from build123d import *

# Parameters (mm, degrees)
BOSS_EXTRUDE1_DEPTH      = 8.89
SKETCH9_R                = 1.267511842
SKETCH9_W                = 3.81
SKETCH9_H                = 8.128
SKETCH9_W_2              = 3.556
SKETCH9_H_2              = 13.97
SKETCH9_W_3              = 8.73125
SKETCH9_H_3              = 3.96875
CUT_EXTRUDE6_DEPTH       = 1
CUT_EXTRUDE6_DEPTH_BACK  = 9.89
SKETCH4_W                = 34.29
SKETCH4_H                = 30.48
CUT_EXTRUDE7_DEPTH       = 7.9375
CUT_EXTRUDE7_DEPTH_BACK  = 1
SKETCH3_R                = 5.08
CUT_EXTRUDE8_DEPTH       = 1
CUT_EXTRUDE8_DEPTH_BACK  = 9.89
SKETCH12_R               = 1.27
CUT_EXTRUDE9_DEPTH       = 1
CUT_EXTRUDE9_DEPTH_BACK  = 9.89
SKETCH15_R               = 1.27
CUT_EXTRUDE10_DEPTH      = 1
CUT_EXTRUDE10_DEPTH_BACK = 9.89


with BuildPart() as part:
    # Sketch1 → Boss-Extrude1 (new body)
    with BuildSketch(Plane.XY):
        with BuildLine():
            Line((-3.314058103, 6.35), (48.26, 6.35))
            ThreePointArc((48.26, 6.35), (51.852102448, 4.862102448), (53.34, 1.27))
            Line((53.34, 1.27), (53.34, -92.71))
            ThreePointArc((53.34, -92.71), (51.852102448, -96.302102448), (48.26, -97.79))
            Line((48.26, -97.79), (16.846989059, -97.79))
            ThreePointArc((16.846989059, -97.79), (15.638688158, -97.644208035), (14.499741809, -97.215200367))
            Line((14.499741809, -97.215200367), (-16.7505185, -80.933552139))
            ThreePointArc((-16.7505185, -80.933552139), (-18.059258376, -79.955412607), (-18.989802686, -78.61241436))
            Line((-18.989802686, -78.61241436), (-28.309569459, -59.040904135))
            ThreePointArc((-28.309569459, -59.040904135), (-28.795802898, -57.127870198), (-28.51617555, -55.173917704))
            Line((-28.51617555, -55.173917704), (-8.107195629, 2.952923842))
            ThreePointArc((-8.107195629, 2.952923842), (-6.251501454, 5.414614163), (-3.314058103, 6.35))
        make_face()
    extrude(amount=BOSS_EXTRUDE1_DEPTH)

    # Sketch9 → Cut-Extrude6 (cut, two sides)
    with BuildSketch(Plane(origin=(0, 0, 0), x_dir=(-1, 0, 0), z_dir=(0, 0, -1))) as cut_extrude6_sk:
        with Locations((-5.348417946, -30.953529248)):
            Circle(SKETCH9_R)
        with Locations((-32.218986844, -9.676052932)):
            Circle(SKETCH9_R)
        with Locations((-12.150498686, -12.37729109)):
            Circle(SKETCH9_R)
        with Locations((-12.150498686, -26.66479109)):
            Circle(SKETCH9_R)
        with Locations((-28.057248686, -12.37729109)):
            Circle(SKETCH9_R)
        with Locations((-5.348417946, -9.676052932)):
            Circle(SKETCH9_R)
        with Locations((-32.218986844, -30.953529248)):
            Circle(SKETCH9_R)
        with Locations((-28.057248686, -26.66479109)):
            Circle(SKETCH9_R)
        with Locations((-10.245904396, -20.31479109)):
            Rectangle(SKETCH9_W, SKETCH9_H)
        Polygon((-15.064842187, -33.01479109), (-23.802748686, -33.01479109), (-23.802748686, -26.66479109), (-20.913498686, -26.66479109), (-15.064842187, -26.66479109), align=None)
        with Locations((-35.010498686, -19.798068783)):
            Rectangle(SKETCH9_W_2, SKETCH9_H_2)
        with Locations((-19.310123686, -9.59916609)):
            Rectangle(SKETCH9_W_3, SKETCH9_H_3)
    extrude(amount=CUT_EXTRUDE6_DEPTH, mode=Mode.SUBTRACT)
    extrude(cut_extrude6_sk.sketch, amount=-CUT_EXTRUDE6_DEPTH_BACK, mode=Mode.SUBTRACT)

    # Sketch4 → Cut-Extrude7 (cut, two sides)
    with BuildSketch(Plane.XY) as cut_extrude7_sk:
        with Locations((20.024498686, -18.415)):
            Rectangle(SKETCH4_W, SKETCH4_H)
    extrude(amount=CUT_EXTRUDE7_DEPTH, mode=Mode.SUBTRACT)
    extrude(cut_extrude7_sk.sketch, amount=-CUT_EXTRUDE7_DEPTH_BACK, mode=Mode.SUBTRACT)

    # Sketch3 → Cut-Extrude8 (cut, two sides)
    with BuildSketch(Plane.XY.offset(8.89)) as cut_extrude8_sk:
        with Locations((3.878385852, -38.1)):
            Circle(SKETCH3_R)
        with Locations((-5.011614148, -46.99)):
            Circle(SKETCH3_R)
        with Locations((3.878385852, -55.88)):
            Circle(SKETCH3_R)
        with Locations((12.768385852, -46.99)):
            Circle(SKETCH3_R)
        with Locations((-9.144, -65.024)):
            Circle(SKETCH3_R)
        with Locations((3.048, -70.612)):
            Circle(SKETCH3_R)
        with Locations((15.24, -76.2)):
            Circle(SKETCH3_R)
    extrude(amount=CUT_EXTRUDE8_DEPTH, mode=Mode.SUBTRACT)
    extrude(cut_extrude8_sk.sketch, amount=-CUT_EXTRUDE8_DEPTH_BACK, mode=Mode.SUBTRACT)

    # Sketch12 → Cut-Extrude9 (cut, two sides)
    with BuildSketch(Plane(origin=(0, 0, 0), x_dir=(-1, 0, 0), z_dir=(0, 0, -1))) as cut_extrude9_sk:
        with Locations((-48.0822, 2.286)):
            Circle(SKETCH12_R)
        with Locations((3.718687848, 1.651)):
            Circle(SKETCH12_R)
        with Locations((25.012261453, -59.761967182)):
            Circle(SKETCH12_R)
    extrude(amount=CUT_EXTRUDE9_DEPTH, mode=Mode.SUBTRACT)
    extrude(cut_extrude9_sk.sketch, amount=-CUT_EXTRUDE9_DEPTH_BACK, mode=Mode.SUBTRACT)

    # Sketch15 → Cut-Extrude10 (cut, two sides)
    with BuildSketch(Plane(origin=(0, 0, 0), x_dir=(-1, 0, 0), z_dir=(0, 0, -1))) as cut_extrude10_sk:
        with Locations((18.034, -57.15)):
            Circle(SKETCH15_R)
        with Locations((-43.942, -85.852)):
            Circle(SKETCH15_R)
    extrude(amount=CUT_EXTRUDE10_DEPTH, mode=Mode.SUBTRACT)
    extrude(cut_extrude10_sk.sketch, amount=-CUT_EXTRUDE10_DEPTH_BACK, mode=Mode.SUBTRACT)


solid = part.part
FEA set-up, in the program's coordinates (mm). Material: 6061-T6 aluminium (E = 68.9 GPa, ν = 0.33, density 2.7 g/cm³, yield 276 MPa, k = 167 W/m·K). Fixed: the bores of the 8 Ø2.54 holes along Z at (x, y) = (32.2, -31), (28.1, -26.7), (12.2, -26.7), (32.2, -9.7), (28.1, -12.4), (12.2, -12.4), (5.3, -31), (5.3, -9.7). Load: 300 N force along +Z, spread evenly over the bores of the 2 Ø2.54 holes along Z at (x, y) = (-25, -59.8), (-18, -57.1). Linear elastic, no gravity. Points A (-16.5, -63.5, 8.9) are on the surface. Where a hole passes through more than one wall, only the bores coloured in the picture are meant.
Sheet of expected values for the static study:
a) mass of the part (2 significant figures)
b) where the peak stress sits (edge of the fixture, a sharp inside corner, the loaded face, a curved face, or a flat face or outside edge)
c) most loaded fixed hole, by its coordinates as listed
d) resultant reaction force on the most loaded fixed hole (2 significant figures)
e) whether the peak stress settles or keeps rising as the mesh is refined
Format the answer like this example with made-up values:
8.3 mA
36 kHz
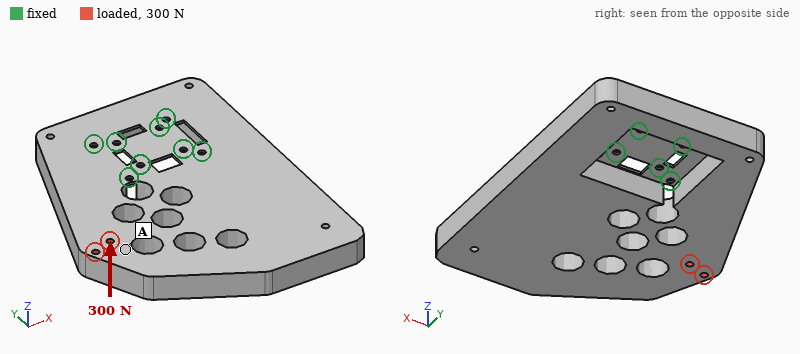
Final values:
140 g
edge of the fixture
(5.3, -31)
750 N
keeps rising
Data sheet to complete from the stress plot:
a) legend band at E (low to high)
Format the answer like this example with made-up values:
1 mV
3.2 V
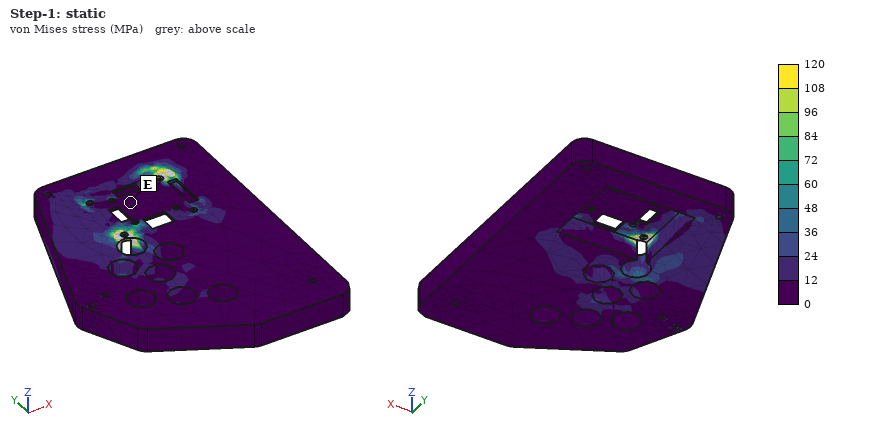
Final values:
0 to 12 MPa
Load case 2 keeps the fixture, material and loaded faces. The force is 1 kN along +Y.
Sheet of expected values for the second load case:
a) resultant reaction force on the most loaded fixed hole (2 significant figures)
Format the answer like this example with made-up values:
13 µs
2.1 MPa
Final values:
800 N
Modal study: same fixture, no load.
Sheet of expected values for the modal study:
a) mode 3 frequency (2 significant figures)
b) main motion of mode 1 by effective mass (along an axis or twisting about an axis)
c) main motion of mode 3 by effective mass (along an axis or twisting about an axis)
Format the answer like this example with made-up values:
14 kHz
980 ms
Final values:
3000 Hz
along Z
along X
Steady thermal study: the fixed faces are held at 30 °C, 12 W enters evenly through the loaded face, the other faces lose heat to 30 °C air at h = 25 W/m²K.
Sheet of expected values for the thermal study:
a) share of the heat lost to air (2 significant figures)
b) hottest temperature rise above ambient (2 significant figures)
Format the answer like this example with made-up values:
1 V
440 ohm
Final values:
23 %
15 K
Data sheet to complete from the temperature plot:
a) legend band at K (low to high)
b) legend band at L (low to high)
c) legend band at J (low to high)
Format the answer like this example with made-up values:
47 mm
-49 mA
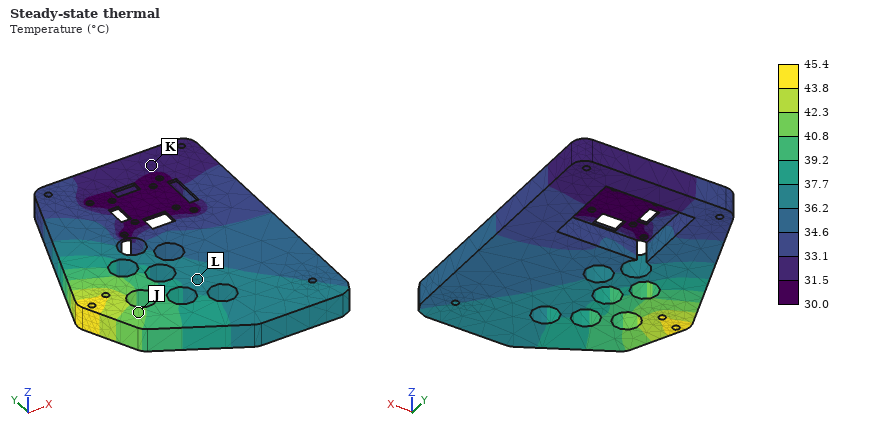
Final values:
31.5 to 33.1 °C
36.2 to 37.7 °C
40.8 to 42.3 °C
